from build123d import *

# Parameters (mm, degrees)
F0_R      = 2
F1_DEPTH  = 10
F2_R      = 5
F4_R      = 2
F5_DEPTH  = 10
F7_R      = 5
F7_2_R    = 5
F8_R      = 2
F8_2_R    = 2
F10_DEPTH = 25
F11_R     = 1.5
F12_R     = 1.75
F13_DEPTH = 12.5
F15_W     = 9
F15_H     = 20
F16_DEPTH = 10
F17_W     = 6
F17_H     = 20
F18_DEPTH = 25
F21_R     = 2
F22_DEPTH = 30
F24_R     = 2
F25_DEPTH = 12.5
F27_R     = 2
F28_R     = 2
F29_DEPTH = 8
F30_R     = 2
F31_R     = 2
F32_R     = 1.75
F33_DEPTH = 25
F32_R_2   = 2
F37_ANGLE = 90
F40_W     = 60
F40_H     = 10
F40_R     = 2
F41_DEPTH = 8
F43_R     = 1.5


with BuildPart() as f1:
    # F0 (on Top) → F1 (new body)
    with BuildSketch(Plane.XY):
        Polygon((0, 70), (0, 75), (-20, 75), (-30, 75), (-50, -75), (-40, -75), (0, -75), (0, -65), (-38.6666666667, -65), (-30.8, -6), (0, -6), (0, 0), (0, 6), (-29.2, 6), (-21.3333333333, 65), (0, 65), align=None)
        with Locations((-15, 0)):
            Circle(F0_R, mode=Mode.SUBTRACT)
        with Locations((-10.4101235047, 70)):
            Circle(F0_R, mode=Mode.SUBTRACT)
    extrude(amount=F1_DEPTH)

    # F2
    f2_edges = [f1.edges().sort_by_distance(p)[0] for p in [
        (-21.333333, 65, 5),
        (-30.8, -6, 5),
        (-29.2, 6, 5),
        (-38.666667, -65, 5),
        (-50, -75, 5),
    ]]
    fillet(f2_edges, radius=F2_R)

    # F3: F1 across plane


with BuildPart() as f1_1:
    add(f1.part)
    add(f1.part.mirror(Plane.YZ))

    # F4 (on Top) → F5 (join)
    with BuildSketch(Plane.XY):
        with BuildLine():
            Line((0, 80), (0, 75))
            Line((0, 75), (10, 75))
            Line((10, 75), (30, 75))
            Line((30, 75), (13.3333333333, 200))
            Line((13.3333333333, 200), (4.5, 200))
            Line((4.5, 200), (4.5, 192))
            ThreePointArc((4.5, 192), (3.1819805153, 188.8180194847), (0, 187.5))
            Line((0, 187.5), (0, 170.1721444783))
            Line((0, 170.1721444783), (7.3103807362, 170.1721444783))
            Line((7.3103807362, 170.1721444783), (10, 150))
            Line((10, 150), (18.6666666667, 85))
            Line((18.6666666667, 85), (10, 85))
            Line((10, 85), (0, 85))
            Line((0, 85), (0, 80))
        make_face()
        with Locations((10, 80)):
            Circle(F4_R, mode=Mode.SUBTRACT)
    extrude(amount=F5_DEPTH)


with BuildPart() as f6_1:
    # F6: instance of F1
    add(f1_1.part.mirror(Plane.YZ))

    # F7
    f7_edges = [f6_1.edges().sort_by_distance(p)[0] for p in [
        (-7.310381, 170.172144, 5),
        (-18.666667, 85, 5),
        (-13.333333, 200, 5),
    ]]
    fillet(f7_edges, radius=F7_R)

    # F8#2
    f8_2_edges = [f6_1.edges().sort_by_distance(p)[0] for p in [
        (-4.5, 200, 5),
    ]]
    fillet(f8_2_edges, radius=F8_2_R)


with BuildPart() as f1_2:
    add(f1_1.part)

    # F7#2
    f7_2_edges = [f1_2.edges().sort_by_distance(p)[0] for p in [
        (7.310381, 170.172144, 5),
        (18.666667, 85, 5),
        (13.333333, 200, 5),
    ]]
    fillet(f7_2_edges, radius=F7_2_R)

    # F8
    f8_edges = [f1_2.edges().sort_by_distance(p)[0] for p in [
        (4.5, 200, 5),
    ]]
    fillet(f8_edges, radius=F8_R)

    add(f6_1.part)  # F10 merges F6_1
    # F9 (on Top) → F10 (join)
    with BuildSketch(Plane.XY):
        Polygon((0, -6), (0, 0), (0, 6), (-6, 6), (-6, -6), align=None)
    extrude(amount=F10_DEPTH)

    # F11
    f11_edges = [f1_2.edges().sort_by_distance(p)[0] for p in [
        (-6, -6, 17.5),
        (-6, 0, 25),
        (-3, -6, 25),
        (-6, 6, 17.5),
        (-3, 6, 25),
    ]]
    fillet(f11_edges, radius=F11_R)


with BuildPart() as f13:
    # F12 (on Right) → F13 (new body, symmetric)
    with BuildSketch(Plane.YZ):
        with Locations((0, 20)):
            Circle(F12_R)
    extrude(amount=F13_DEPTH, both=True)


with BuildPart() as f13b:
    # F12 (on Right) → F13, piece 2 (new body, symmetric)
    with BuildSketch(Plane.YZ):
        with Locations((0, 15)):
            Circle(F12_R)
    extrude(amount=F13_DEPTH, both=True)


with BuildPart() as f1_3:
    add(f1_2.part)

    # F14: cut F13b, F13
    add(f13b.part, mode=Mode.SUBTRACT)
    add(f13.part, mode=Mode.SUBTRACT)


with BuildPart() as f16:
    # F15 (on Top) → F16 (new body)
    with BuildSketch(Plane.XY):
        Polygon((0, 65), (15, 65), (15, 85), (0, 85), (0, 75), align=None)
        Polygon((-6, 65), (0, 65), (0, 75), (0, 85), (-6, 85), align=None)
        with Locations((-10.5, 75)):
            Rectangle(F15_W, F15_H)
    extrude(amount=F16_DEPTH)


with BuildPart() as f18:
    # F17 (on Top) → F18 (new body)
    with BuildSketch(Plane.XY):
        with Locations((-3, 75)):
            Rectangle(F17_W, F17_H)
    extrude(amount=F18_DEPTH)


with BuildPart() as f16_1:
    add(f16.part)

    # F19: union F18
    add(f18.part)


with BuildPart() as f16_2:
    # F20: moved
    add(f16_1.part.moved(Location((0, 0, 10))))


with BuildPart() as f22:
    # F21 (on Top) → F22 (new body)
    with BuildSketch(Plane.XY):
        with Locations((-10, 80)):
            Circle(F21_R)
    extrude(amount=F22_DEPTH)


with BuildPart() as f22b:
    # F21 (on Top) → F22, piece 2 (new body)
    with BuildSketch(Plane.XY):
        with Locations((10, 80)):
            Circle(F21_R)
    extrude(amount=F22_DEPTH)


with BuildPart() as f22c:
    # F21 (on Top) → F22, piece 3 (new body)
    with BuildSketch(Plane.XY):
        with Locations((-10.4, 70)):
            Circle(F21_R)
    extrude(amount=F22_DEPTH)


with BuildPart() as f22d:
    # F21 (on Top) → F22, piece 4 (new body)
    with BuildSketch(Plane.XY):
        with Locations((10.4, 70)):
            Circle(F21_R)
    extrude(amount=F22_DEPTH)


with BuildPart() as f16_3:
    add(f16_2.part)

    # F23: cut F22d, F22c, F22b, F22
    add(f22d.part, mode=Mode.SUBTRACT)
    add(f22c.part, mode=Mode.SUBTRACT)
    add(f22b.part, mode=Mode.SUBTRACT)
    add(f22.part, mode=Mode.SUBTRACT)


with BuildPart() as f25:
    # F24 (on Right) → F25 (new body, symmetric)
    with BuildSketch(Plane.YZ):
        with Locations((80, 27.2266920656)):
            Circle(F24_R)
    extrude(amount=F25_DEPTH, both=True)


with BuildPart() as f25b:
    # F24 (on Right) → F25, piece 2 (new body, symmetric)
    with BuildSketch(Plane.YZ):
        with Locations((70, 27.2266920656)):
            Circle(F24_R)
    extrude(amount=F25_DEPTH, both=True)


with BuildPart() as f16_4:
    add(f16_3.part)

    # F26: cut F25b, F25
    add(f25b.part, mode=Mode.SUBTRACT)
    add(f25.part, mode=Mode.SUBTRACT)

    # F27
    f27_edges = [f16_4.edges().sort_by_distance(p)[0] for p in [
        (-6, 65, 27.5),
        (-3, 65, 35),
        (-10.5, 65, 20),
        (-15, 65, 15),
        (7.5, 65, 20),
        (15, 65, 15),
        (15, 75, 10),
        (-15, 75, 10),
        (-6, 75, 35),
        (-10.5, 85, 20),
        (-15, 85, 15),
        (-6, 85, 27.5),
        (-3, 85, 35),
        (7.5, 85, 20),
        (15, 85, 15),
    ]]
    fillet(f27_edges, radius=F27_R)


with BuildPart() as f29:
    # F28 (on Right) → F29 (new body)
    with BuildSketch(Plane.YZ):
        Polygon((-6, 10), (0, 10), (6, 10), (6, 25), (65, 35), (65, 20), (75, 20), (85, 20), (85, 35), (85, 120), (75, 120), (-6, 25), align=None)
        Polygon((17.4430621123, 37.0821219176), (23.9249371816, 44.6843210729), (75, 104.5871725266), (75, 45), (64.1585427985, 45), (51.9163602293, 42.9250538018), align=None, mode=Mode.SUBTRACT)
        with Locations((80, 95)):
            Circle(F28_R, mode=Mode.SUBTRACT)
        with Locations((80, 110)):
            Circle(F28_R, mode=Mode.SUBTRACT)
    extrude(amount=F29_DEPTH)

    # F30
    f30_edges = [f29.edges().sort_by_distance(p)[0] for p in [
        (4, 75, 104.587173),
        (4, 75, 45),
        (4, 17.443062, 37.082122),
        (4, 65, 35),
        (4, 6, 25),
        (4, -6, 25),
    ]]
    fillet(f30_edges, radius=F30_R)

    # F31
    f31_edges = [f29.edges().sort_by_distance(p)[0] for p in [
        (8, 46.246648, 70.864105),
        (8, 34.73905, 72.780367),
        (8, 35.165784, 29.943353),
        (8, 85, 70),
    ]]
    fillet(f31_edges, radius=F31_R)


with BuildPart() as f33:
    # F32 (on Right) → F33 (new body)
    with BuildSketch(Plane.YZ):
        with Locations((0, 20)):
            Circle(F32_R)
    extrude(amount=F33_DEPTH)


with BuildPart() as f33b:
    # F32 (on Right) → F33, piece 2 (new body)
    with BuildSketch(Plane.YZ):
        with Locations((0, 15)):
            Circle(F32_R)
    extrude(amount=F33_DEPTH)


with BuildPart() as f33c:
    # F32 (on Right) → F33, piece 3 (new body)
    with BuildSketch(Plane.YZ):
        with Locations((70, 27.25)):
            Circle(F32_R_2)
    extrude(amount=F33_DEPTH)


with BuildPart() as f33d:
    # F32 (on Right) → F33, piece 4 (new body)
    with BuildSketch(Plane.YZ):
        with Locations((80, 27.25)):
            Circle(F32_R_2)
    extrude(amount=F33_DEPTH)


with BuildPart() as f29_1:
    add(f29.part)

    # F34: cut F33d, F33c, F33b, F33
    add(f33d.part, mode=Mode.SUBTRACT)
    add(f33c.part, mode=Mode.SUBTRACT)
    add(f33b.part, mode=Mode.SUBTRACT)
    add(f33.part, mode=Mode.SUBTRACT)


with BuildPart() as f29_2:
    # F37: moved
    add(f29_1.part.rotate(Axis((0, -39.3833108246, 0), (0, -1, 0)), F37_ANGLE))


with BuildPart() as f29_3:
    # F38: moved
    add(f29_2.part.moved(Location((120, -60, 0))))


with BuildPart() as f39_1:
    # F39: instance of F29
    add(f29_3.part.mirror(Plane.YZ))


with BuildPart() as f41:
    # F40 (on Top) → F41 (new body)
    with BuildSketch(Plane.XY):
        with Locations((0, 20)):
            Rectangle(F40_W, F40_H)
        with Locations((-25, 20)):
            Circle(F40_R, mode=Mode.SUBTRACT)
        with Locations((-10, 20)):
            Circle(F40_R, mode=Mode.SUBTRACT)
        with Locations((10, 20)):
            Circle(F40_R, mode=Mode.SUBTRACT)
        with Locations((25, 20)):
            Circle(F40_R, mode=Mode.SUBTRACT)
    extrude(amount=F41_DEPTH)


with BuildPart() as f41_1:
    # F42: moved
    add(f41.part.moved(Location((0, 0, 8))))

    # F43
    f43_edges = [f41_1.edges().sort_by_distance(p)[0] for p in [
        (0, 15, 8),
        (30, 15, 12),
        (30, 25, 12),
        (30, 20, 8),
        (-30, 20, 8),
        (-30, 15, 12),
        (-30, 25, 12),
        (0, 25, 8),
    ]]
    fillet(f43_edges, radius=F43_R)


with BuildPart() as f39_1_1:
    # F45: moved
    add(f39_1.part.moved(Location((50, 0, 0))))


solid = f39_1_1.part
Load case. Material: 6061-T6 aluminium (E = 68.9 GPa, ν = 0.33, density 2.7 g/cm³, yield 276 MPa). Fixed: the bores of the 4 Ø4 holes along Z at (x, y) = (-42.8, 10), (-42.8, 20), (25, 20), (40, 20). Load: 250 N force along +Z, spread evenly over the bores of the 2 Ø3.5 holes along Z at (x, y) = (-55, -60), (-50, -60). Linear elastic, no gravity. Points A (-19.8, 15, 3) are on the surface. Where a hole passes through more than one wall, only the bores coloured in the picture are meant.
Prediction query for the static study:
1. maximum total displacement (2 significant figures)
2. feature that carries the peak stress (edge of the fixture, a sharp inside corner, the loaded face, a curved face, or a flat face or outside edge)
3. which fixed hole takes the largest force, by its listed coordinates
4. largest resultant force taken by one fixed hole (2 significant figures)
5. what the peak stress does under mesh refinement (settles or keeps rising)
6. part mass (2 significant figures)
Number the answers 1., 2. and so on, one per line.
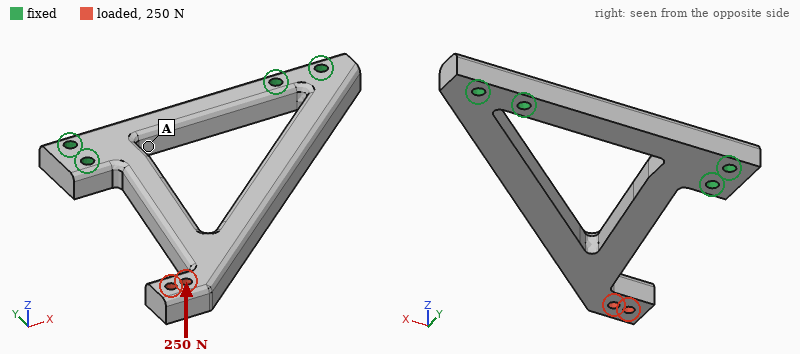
1. 1.1 mm
2. a sharp inside corner
3. (-42.8, 10)
4. 960 N
5. keeps rising
6. 65 g
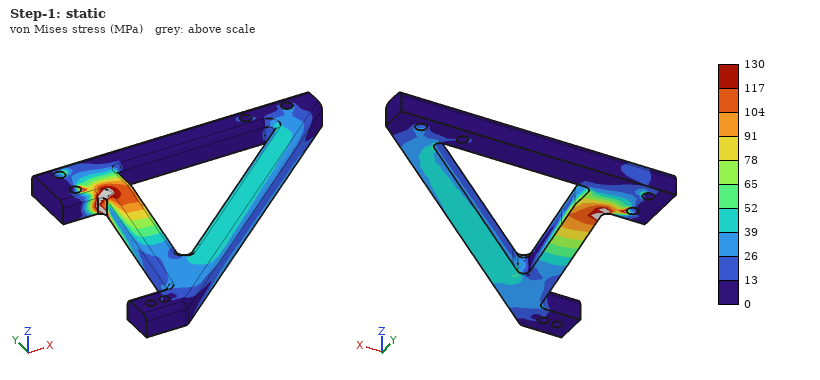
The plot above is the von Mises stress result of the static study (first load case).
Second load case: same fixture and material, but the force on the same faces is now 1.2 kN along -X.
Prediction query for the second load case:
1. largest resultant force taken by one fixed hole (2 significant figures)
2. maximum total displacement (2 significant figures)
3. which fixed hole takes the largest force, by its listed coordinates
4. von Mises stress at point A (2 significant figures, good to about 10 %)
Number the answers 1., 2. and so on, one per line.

1. 1.9 kN
2. 0.17 mm
3. (40, 20)
4. 6.1 MPa
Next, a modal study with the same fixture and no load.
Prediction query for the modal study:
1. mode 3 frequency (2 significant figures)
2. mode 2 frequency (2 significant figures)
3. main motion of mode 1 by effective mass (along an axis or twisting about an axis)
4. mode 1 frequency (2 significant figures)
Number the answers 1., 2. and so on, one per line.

1. 4000 Hz
2. 2800 Hz
3. along Z
4. 840 Hz
